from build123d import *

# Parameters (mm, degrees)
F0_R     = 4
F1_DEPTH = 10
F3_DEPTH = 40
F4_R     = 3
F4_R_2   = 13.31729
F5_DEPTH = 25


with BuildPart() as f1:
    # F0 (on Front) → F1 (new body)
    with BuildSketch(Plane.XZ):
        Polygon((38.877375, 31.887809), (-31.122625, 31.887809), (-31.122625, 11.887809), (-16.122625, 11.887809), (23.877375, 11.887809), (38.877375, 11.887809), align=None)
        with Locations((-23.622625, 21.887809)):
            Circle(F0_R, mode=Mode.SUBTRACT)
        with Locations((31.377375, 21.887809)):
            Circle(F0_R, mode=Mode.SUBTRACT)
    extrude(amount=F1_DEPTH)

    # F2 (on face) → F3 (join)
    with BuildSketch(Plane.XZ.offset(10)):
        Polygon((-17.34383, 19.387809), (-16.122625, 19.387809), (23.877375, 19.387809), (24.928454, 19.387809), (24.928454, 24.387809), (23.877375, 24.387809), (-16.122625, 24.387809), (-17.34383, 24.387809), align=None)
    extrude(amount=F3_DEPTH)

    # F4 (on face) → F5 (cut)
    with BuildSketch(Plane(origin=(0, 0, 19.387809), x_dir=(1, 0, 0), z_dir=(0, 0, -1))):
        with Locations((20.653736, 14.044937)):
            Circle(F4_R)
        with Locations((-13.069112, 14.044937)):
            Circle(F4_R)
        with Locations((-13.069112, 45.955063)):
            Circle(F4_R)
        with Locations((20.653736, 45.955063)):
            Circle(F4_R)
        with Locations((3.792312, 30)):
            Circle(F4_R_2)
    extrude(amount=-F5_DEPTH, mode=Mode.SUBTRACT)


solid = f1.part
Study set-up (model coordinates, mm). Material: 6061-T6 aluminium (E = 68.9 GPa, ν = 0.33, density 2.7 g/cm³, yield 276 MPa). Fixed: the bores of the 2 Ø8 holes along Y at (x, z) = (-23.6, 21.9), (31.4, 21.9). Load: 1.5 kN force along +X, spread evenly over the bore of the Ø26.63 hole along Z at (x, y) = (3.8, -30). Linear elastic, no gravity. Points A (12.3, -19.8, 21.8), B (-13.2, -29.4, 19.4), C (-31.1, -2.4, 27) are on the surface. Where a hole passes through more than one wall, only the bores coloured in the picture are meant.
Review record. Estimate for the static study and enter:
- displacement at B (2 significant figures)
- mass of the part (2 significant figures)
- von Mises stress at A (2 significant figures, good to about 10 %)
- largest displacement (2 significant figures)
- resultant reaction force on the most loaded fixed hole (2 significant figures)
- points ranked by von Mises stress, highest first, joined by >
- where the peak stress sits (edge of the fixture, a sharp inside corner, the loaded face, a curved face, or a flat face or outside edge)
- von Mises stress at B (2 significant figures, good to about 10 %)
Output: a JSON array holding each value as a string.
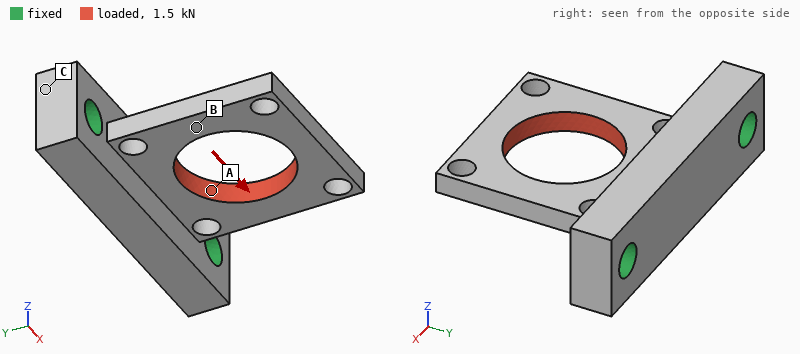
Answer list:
["34 µm", "49 g", "66 MPa", "69 µm", "1.1 kN", "A > B > C", "a curved face", "26 MPa"]
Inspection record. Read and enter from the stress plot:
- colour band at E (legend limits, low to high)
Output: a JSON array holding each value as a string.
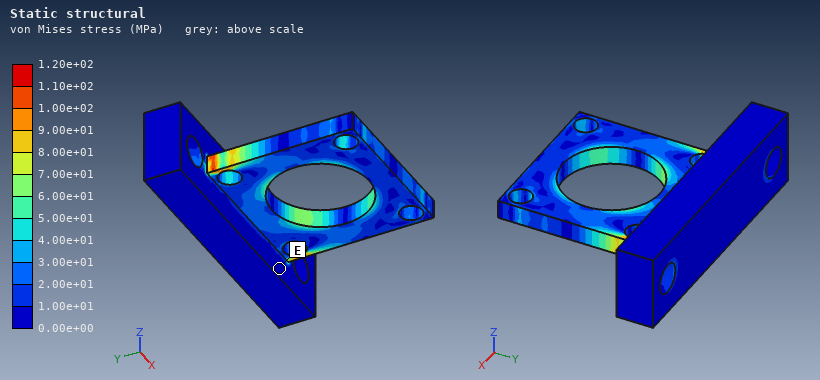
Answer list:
["0.00e+00 to 1.00e+01 MPa"]
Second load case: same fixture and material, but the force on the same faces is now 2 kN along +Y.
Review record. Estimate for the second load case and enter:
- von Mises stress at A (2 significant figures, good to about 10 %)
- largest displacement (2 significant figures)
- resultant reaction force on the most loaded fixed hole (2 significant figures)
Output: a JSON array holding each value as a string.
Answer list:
["13 MPa", "22 µm", "1.0 kN"]
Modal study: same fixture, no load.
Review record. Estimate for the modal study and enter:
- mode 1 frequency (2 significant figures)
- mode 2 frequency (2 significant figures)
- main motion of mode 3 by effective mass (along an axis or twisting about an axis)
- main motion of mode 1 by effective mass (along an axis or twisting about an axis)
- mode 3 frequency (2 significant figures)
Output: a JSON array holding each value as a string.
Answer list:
["1900 Hz", "4300 Hz", "along X", "along Z", "7000 Hz"]
